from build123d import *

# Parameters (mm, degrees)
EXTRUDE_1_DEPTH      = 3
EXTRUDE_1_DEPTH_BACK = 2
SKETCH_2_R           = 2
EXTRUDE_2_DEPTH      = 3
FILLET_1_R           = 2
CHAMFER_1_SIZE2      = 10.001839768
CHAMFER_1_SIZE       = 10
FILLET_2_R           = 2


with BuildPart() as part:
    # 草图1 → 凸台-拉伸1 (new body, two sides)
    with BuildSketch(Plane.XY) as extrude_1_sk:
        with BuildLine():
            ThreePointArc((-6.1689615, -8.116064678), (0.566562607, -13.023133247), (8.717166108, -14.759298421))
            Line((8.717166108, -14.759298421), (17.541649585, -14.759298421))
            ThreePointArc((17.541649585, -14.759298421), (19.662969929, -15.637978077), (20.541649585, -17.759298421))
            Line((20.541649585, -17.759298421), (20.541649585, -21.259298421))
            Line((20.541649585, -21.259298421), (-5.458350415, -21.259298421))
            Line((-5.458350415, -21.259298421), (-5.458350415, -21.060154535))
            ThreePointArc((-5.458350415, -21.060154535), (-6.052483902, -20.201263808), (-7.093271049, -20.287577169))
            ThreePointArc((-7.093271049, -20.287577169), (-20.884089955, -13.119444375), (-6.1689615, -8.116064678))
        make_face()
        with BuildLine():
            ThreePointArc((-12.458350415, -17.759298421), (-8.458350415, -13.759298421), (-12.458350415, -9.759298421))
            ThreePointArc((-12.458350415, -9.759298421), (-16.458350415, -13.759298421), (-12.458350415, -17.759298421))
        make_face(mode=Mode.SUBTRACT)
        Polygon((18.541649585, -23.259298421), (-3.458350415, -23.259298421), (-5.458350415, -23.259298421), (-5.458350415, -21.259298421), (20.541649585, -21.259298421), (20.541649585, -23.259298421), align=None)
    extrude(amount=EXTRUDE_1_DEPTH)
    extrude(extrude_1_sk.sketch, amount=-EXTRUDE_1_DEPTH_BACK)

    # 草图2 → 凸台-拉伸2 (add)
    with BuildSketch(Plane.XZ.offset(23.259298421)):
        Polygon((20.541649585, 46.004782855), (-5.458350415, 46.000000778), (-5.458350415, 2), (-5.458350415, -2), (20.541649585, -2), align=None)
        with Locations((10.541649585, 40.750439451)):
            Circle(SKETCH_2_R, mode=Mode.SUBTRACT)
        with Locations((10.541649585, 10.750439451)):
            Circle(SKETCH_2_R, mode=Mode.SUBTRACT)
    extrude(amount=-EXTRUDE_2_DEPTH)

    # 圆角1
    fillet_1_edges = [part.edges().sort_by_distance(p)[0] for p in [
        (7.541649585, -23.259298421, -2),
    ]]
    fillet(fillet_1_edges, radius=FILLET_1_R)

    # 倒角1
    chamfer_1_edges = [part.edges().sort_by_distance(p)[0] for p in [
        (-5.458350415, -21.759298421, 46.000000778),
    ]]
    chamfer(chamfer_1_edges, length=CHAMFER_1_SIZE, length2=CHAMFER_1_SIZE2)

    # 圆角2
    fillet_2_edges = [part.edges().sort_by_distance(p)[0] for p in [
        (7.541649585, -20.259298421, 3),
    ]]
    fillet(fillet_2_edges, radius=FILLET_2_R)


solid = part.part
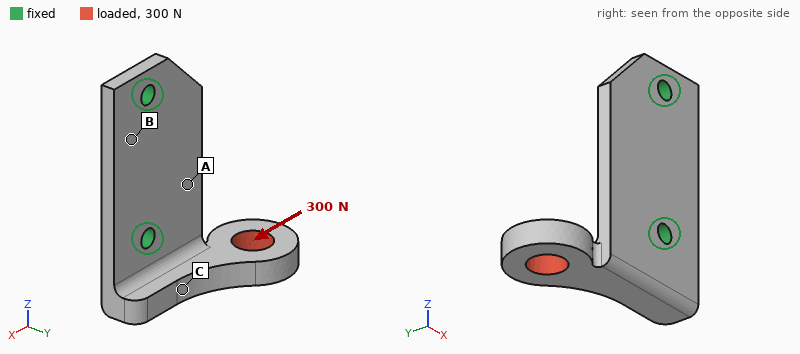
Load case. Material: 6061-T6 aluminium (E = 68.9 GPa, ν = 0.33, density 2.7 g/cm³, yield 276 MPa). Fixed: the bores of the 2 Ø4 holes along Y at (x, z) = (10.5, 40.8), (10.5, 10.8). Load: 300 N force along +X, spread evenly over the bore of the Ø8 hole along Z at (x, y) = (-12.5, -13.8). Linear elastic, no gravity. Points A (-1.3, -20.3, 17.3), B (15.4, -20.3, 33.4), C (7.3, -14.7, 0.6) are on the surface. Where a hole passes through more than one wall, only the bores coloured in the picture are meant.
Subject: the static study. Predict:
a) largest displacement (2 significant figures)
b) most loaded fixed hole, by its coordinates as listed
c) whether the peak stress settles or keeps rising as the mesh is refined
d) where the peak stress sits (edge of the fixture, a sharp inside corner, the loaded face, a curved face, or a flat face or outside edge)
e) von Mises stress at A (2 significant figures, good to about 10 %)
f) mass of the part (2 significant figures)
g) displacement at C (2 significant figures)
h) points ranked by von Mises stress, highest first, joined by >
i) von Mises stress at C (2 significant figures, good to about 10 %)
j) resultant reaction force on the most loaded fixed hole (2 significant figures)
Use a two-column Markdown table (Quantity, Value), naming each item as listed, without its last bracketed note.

| Quantity | Value |
|---|---|
| largest displacement | 0.11 mm |
| most loaded fixed hole, by its coordinates as listed | (10.5, 10.8) |
| whether the peak stress settles or keeps rising as the mesh is refined | keeps rising |
| where the peak stress sits | edge of the fixture |
| von Mises stress at A | 15 MPa |
| mass of the part | 14 g |
| displacement at C | 0.024 mm |
| points ranked by von Mises stress, highest first, joined by > | C > A > B |
| von Mises stress at C | 27 MPa |
| resultant reaction force on the most loaded fixed hole | 380 N |
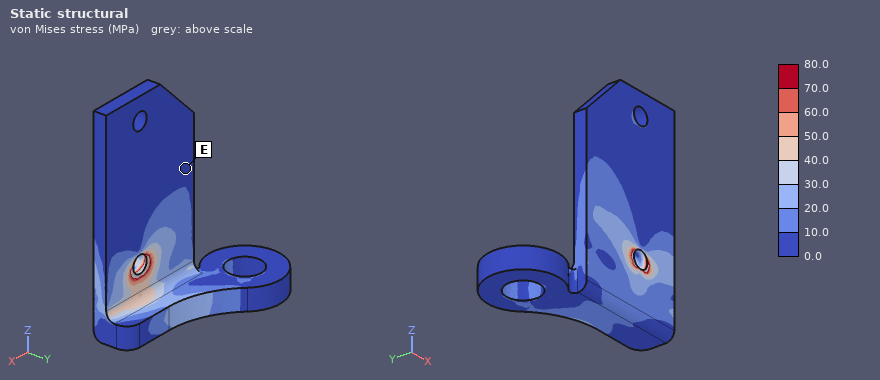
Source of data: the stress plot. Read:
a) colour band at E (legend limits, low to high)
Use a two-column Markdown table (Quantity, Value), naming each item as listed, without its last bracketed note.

| Quantity | Value |
|---|---|
| colour band at E | 0.0 to 10.0 MPa |
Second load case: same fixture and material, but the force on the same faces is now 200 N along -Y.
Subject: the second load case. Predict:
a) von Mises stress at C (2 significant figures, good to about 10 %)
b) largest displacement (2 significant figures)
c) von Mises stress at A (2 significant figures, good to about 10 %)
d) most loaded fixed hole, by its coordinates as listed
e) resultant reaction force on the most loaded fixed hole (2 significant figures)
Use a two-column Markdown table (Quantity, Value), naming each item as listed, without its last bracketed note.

| Quantity | Value |
|---|---|
| von Mises stress at C | 45 MPa |
| largest displacement | 0.24 mm |
| von Mises stress at A | 41 MPa |
| most loaded fixed hole, by its coordinates as listed | (10.5, 10.8) |
| resultant reaction force on the most loaded fixed hole | 220 N |
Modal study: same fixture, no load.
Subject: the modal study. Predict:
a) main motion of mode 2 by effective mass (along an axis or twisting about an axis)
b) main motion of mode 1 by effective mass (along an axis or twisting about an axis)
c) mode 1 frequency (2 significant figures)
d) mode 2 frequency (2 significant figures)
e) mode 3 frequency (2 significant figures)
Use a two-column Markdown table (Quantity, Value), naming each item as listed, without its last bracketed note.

| Quantity | Value |
|---|---|
| main motion of mode 2 by effective mass | along Z |
| main motion of mode 1 by effective mass | along Y |
| mode 1 frequency | 3000 Hz |
| mode 2 frequency | 5000 Hz |
| mode 3 frequency | 9100 Hz |
